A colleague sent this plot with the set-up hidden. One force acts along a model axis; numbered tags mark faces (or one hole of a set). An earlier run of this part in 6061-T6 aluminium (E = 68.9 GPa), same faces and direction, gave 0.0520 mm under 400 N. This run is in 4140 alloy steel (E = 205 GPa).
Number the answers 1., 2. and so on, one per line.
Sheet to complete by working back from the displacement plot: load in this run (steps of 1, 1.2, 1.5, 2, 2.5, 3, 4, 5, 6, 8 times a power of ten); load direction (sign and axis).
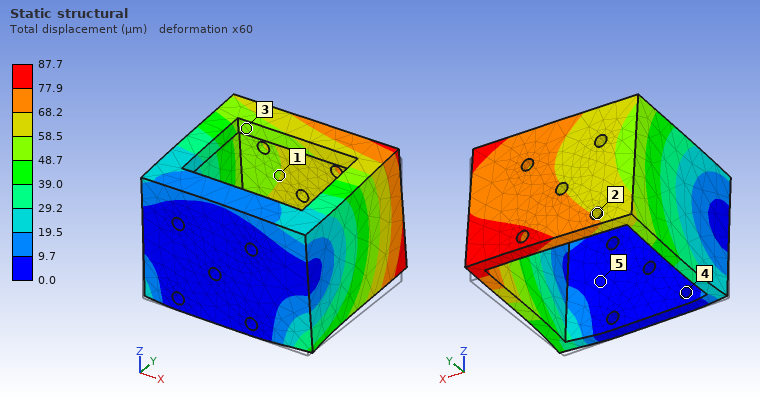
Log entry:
1. 2 kN
2. +Z
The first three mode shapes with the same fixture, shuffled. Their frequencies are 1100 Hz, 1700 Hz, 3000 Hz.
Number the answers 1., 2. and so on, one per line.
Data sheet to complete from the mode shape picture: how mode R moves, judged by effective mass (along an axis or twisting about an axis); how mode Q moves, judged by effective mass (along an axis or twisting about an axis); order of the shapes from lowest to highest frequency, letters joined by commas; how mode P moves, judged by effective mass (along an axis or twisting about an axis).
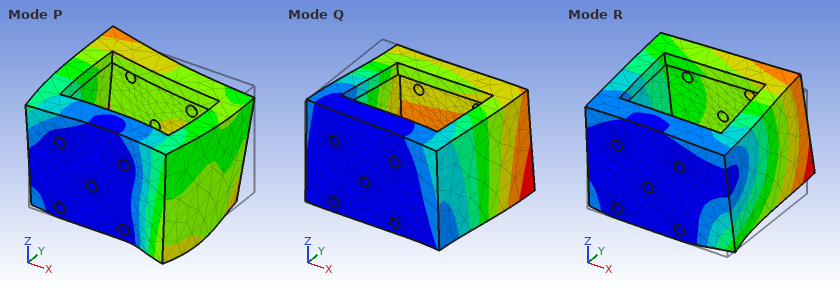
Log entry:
1. along Z
2. along X
3. Q, R, P
4. along Y
